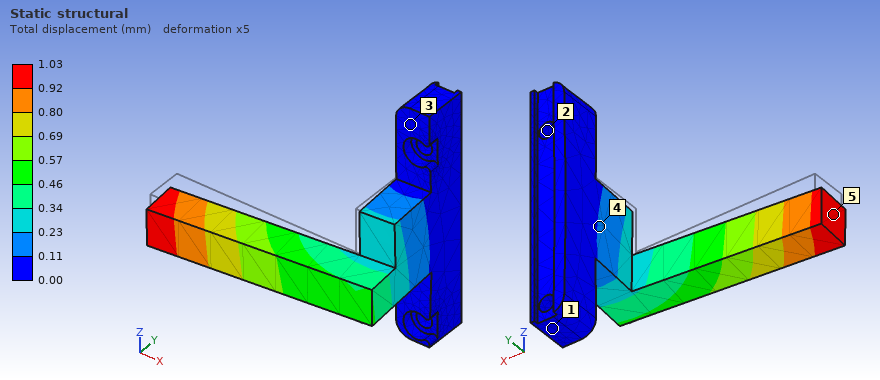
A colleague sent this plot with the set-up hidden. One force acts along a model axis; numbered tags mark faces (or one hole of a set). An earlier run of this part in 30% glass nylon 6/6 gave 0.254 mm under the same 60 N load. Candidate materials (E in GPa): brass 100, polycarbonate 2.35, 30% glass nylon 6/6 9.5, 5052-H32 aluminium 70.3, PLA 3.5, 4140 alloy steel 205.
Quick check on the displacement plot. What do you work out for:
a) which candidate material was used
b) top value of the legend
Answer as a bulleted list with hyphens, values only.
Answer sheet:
- polycarbonate
- 1.03 mm
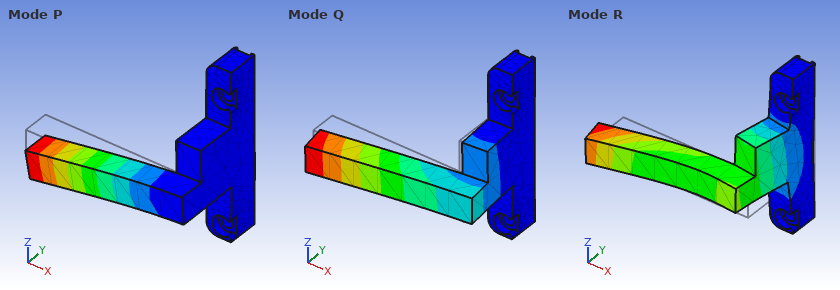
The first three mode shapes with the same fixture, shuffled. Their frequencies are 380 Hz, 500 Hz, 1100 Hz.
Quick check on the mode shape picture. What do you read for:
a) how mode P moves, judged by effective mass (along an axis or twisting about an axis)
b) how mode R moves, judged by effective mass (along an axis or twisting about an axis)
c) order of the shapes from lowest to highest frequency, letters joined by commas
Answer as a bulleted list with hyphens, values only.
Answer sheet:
- along Z
- along X
- Q, P, R
